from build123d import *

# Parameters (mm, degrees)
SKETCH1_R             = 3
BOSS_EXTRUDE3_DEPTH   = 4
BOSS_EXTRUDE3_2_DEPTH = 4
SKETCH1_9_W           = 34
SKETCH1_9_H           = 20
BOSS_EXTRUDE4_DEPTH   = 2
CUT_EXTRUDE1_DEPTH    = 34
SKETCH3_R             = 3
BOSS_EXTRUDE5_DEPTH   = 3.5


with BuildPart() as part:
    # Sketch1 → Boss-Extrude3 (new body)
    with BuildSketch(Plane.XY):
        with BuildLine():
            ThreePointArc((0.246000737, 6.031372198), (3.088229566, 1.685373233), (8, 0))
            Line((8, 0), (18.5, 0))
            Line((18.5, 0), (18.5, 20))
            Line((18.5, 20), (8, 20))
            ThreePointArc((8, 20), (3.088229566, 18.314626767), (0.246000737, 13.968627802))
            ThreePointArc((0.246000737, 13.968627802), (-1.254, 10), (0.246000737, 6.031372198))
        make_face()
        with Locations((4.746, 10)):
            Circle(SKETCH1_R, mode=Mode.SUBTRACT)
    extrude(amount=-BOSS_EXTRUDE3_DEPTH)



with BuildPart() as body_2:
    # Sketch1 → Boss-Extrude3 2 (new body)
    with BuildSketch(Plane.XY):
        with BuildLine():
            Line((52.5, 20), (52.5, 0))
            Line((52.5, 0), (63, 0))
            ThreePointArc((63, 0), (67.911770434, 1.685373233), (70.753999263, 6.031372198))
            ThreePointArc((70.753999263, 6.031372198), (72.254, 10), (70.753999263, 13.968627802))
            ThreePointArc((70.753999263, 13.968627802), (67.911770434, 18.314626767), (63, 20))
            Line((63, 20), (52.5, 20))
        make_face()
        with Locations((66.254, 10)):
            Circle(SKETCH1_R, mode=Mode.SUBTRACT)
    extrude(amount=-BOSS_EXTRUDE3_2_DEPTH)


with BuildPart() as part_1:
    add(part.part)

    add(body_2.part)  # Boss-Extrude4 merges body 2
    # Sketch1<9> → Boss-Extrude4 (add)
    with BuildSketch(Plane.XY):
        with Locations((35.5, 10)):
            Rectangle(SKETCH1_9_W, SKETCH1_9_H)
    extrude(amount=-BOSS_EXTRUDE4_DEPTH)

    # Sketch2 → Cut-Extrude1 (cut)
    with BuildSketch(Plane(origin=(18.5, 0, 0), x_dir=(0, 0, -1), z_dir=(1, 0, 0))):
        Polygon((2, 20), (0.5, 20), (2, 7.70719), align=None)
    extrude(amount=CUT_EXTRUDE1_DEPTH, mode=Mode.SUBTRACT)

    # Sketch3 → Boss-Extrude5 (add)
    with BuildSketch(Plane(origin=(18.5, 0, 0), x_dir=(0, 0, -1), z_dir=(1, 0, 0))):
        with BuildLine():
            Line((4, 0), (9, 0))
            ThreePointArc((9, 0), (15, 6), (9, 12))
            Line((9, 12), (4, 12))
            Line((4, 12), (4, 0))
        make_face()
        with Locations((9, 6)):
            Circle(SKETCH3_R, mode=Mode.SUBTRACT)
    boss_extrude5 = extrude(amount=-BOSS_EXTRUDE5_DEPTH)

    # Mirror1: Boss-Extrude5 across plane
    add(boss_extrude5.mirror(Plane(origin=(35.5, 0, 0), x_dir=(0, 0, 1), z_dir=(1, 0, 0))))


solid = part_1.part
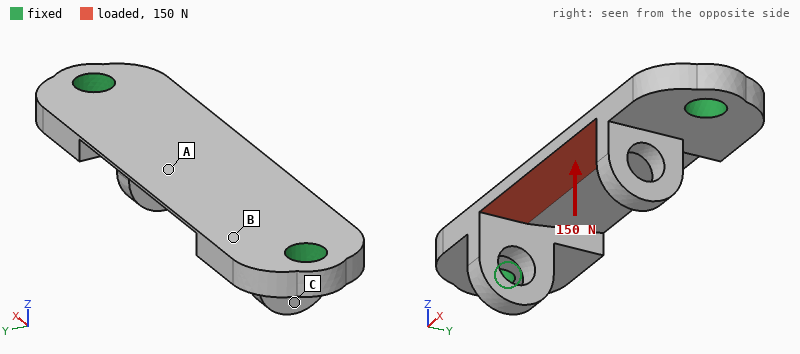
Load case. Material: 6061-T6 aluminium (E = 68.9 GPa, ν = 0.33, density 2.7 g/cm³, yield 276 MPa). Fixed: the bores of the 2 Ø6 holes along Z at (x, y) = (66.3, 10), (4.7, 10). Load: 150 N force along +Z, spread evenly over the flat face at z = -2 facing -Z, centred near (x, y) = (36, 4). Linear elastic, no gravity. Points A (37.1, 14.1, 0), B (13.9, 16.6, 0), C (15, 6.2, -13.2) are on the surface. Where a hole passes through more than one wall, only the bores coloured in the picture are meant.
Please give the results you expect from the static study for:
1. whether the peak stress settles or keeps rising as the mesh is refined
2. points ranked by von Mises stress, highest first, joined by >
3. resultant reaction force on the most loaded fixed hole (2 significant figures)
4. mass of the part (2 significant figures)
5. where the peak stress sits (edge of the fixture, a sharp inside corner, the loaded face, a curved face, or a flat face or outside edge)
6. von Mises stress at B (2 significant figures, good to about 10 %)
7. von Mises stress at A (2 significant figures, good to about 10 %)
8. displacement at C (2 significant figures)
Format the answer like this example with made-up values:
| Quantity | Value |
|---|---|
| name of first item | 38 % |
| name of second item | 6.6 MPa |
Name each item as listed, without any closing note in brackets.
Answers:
| Quantity | Value |
|---|---|
| whether the peak stress settles or keeps rising as the mesh is refined | keeps rising |
| points ranked by von Mises stress, highest first, joined by > | A > B > C |
| resultant reaction force on the most loaded fixed hole | 140 N |
| mass of the part | 11 g |
| where the peak stress sits | edge of the fixture |
| von Mises stress at B | 9.3 MPa |
| von Mises stress at A | 20 MPa |
| displacement at C | 18 µm |
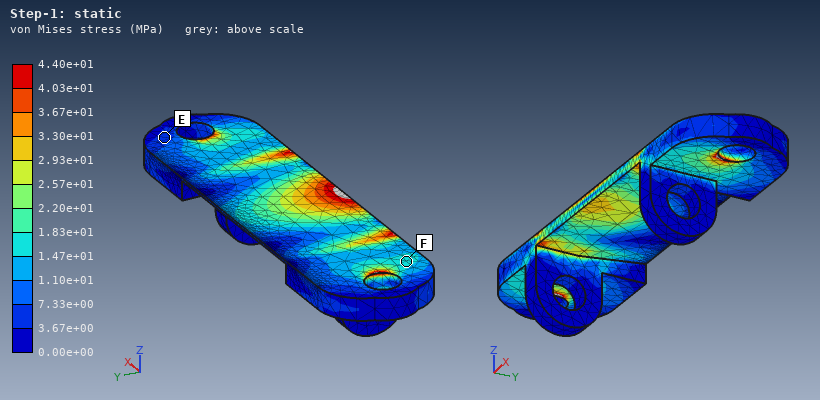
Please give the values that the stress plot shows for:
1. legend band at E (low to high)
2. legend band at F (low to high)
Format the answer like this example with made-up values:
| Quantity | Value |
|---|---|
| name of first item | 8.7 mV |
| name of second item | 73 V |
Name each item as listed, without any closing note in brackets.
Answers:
| Quantity | Value |
|---|---|
| legend band at E | 3.67e+00 to 7.33e+00 MPa |
| legend band at F | 1.47e+01 to 1.83e+01 MPa |
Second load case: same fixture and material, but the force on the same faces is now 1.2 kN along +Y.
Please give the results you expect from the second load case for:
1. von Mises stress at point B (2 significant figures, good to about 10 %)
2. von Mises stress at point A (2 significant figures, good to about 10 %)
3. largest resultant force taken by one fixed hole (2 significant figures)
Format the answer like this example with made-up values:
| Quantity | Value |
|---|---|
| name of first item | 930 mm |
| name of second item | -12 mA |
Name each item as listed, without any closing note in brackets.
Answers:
| Quantity | Value |
|---|---|
| von Mises stress at point B | 17 MPa |
| von Mises stress at point A | 36 MPa |
| largest resultant force taken by one fixed hole | 620 N |
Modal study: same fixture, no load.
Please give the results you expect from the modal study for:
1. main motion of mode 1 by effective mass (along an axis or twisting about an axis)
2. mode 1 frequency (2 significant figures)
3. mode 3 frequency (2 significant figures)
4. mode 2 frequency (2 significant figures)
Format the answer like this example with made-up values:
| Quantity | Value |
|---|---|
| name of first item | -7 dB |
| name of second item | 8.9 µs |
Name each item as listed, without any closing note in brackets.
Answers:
| Quantity | Value |
|---|---|
| main motion of mode 1 by effective mass | along Z |
| mode 1 frequency | 5400 Hz |
| mode 3 frequency | 9600 Hz |
| mode 2 frequency | 8600 Hz |
